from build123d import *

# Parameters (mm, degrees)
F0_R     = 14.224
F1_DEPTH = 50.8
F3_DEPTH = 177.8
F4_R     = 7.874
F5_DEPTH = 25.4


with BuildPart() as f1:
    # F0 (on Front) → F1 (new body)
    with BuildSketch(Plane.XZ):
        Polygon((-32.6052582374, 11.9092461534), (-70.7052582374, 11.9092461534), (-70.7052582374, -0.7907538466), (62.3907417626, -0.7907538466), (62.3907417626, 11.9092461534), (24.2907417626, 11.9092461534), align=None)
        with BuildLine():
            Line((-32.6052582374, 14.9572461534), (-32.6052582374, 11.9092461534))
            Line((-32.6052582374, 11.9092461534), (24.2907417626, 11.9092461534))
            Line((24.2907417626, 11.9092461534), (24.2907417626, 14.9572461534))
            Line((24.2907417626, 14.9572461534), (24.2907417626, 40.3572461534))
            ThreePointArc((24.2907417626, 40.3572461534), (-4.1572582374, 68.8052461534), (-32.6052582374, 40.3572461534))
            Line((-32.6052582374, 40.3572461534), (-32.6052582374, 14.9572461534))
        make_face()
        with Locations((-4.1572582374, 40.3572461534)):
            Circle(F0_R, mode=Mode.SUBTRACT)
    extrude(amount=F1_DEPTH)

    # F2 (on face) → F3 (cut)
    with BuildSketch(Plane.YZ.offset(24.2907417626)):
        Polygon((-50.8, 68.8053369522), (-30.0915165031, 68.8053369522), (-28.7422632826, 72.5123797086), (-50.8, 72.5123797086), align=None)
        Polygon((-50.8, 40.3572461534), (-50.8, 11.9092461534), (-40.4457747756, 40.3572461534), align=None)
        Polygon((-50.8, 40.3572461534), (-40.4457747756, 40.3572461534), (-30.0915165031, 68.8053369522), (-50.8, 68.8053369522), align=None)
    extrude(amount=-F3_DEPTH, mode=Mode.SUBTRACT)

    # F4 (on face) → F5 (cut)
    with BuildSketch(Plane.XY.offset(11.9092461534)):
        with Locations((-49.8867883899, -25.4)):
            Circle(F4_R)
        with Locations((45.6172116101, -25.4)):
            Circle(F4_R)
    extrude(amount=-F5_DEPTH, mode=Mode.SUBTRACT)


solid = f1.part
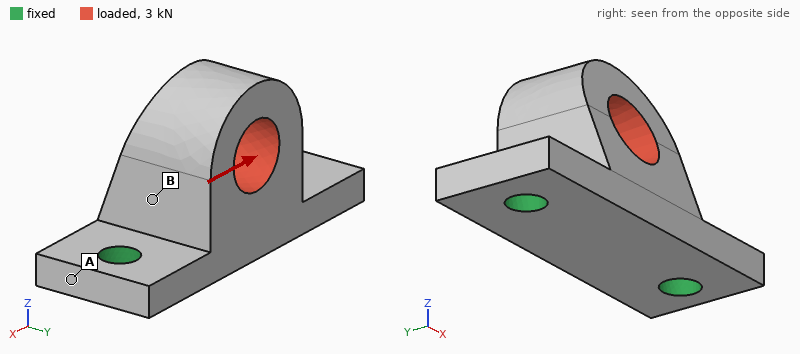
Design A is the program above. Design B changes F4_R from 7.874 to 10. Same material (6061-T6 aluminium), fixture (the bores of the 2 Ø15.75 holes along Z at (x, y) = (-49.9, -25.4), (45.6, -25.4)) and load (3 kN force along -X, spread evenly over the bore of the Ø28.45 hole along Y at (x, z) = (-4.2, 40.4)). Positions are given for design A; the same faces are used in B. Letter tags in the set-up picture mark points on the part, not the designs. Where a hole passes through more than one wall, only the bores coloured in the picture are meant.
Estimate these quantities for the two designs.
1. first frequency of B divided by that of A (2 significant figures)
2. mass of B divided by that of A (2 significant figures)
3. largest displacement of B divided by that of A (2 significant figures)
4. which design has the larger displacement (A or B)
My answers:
1.1
0.98
0.89
A
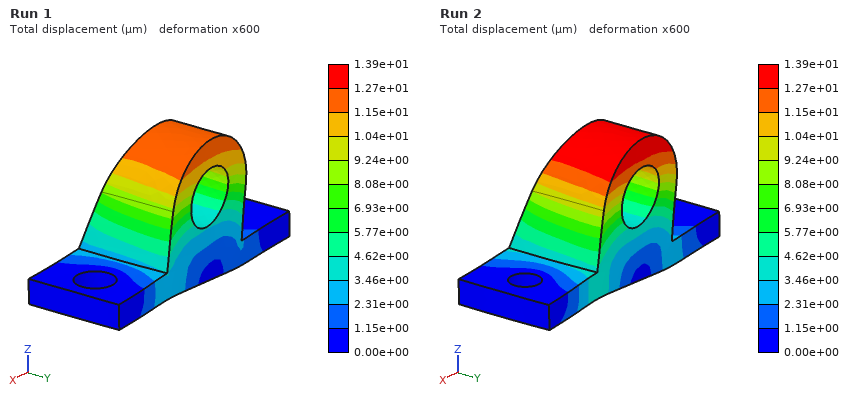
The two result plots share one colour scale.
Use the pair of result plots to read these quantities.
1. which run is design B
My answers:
Run 1
